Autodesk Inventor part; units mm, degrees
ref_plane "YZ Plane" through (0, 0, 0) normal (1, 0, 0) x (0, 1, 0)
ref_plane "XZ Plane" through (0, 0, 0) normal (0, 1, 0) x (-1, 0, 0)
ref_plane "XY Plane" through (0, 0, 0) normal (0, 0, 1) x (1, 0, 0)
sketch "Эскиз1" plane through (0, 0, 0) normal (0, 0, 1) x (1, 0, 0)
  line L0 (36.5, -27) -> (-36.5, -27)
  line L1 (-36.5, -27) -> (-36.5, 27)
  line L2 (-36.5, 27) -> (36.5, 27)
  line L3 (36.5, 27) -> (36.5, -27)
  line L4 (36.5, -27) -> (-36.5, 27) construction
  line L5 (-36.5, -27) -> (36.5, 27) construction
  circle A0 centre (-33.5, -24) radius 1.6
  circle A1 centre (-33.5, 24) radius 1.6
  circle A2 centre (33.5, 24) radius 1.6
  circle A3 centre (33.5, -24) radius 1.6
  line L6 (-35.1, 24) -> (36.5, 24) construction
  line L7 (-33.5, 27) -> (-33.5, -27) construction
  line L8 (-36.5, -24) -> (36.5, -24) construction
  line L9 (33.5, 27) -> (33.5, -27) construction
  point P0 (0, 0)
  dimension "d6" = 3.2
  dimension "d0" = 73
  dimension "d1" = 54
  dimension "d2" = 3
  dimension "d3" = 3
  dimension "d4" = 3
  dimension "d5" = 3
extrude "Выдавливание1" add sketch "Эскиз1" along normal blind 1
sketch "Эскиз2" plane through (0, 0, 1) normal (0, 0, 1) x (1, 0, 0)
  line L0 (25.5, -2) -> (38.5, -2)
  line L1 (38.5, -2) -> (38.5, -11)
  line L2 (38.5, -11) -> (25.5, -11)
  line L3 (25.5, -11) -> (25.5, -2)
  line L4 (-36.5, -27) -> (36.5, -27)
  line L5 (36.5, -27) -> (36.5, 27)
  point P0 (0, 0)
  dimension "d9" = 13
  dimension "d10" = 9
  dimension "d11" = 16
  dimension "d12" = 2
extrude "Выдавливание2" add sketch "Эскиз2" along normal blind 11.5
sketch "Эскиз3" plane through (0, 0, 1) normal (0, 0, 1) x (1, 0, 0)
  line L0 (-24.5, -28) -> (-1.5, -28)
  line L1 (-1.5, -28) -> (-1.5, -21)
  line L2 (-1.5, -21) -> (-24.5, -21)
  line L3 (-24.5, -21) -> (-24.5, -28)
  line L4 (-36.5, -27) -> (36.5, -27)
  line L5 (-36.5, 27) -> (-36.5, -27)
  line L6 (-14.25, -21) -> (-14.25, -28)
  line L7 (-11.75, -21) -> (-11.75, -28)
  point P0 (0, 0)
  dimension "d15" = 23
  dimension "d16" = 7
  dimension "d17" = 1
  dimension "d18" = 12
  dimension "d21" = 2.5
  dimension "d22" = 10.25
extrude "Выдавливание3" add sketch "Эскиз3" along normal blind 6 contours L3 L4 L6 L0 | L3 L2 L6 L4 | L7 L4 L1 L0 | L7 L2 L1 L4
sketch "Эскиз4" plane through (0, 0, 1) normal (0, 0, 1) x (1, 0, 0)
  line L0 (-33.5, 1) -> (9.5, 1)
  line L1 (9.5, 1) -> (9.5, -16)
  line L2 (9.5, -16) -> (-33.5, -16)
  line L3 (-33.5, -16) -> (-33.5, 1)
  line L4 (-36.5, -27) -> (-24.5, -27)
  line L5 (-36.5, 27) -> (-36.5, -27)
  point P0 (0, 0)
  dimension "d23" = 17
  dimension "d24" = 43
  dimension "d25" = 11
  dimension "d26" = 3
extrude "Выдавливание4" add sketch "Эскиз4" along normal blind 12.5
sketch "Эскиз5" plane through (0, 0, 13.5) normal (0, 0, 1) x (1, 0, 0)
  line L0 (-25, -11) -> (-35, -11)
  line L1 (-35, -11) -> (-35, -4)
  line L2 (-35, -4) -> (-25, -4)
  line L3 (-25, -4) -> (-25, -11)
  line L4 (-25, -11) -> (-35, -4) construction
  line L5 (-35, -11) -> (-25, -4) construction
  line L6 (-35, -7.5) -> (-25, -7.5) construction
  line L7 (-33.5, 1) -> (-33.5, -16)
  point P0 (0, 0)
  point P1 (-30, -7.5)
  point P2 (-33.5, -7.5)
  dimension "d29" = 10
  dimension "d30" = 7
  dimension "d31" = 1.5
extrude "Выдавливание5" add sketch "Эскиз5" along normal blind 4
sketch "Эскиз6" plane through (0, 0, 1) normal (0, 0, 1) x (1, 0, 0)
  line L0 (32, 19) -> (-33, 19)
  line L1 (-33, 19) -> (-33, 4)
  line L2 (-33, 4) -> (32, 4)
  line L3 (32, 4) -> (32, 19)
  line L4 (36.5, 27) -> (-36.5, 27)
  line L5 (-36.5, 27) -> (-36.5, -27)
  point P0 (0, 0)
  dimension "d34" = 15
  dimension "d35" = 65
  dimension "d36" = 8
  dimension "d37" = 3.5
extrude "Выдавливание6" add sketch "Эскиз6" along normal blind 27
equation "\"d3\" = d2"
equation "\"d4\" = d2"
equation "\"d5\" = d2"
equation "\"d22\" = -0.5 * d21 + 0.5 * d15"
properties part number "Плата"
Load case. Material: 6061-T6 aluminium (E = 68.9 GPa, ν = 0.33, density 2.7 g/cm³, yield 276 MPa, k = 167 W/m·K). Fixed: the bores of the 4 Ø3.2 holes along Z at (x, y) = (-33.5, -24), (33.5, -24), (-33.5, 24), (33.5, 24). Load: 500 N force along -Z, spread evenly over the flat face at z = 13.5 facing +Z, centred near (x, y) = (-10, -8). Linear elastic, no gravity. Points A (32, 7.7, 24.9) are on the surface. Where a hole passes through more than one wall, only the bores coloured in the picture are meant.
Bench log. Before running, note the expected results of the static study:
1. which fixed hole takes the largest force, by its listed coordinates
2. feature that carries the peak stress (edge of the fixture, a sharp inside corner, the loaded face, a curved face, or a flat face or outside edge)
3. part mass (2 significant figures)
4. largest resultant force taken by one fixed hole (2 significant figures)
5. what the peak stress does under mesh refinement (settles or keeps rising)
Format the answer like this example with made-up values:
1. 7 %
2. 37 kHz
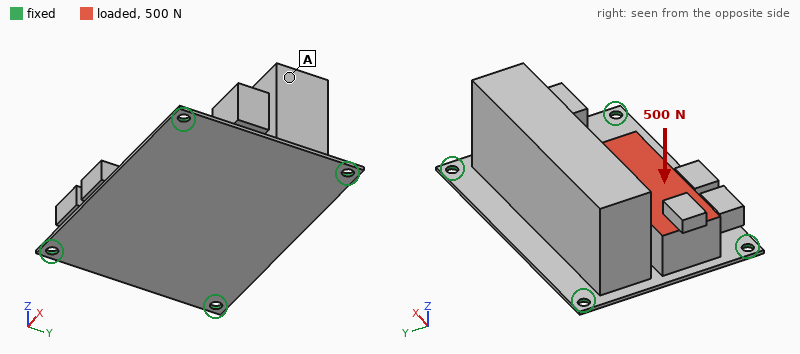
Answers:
1. (-33.5, -24)
2. edge of the fixture
3. 110 g
4. 340 N
5. keeps rising
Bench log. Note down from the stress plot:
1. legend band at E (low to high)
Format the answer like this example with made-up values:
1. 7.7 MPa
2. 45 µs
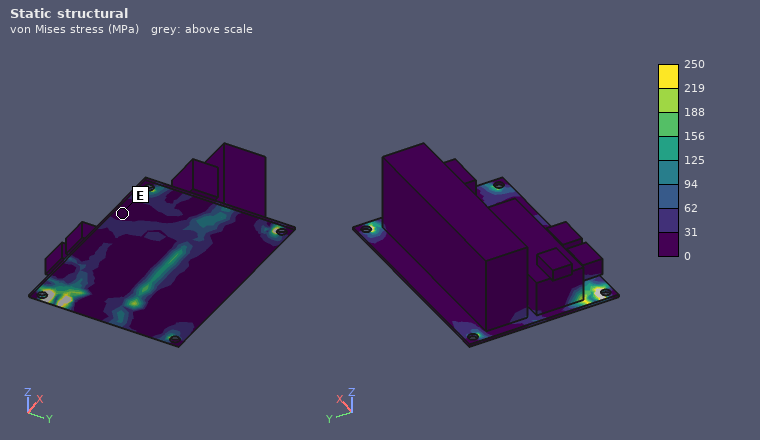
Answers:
1. 0 to 31 MPa
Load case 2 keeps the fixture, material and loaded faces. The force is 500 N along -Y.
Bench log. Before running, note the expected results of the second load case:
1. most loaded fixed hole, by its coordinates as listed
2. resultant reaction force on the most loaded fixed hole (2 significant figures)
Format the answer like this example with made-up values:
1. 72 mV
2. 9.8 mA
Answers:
1. (-33.5, 24)
2. 290 N
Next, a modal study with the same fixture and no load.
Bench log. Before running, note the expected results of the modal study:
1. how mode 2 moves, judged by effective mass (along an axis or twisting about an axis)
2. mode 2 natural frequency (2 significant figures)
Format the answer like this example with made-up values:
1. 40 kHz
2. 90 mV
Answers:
1. along Z
2. 1800 Hz
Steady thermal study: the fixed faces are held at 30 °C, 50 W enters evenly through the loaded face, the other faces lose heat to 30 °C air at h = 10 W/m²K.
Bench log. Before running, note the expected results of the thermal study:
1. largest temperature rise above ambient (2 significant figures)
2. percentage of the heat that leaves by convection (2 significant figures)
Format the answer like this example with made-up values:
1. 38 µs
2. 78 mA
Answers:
1. 69 K
2. 13 %
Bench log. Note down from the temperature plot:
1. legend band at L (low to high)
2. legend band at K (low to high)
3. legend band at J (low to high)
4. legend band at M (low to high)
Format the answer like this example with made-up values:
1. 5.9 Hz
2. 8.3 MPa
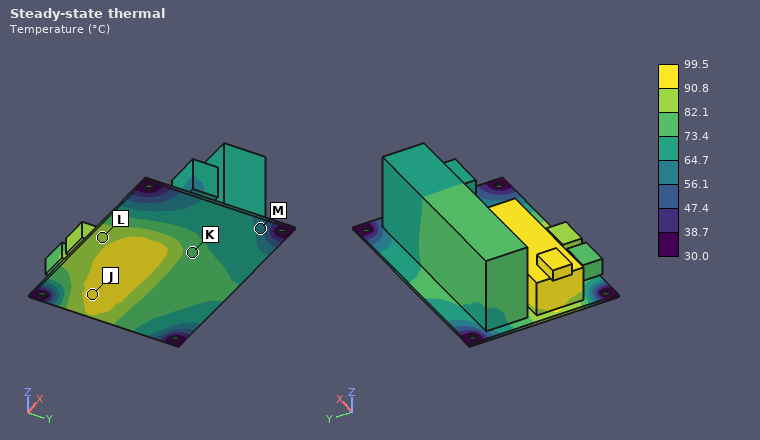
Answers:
1. 82.1 to 90.8 °C
2. 73.4 to 82.1 °C
3. 90.8 to 99.5 °C
4. 56.1 to 64.7 °C
